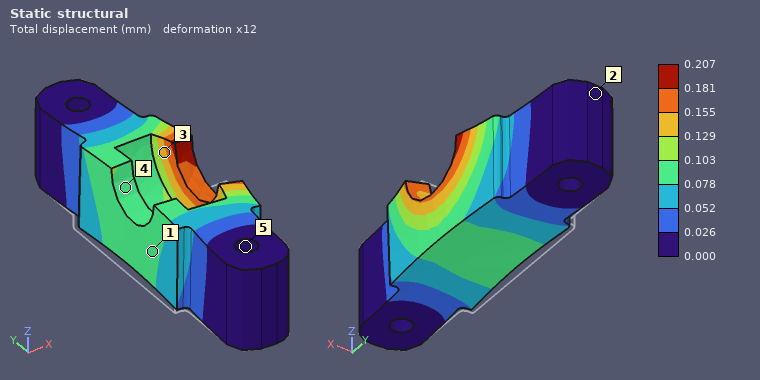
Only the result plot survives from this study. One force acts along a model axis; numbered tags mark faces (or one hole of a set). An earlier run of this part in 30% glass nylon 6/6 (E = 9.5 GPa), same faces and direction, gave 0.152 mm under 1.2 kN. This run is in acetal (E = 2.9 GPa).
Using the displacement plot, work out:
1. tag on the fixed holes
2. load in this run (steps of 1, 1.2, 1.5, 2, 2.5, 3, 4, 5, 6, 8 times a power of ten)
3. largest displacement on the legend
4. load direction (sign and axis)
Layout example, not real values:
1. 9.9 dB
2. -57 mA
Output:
1. 5
2. 500 N
3. 0.207 mm
4. +X
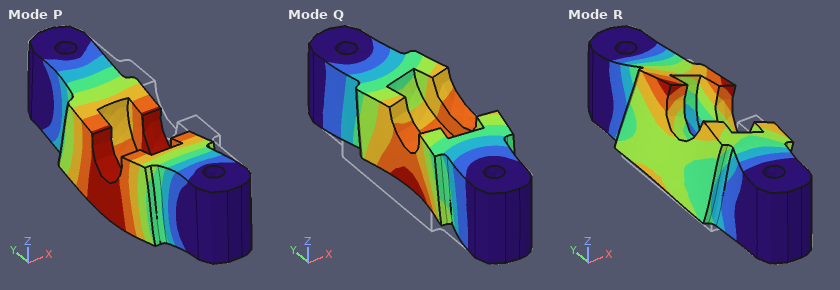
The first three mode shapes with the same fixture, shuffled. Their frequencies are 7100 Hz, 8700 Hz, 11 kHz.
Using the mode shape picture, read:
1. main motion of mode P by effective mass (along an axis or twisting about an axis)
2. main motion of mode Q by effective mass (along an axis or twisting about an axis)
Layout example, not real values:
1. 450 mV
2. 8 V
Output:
1. along Z
2. along X
